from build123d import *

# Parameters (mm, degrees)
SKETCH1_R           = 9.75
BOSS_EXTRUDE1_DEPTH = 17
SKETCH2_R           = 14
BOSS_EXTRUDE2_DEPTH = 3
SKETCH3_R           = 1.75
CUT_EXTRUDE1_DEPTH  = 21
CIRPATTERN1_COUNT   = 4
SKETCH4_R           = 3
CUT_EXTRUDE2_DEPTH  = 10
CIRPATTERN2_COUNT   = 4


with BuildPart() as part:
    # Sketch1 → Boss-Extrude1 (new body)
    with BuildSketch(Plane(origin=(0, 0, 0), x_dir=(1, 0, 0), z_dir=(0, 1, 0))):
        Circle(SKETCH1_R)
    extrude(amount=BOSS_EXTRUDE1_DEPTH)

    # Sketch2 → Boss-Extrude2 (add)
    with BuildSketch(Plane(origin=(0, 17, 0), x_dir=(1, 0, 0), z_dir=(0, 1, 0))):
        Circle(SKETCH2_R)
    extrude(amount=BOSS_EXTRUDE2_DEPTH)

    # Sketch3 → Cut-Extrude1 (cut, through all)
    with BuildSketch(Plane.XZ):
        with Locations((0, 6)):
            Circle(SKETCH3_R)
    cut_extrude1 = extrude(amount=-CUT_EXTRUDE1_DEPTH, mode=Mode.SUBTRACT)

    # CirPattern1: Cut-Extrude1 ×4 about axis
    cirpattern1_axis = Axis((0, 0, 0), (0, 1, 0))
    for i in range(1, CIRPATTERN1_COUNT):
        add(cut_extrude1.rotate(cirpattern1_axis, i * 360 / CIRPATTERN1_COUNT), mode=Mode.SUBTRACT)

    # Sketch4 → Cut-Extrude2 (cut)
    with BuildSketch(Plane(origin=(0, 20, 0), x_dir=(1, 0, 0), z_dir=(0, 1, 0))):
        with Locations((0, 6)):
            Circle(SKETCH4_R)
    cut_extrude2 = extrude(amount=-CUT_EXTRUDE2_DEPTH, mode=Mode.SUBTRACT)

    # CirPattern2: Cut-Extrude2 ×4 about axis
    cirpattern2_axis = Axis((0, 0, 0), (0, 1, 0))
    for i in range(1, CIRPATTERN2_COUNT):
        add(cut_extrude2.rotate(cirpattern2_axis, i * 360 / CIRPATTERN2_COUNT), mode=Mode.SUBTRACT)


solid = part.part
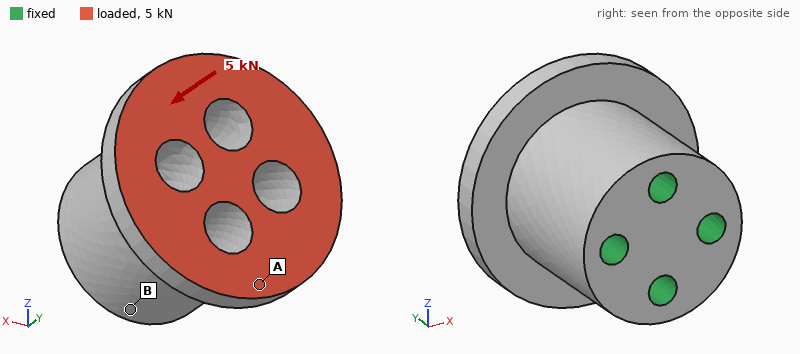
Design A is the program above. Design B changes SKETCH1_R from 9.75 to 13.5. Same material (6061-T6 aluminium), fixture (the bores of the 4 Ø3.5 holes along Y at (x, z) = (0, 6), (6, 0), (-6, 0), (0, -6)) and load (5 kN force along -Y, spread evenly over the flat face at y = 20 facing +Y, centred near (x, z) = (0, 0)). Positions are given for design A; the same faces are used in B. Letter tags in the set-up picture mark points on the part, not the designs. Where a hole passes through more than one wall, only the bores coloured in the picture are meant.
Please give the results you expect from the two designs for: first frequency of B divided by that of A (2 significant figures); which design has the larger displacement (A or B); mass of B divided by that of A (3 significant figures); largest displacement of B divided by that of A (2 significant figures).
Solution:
1.2
A
1.86
0.16
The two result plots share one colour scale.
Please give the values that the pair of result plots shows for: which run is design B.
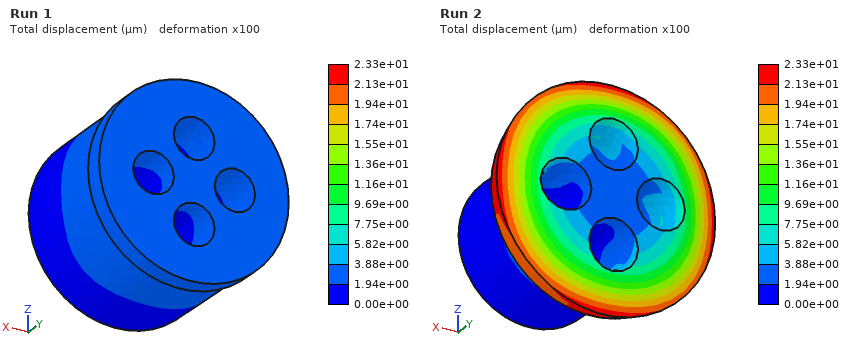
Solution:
Run 1
